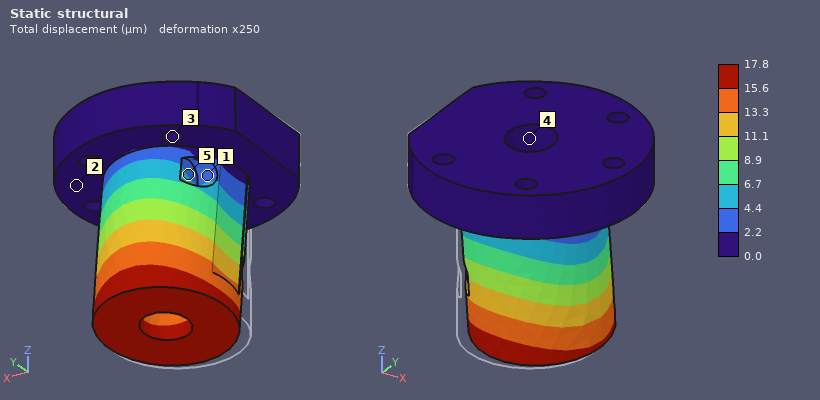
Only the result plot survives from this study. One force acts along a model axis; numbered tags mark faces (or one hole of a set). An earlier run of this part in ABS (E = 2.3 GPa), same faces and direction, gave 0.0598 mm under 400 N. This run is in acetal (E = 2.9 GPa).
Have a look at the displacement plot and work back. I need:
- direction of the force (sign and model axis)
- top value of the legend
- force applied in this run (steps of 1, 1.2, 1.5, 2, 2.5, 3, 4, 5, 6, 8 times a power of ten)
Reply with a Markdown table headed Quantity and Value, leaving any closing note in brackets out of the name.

| Quantity | Value |
|---|---|
| direction of the force | +Y |
| top value of the legend | 17.8 µm |
| force applied in this run | 150 N |
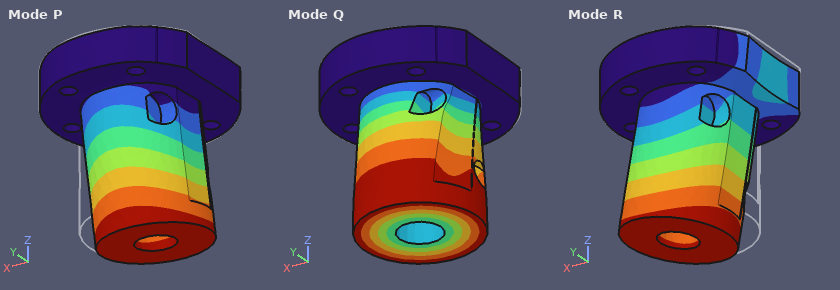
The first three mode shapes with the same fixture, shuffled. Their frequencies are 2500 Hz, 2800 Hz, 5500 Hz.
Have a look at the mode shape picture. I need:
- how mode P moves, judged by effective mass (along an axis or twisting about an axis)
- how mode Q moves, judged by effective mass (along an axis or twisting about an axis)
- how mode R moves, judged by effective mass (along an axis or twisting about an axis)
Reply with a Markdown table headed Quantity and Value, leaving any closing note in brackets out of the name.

| Quantity | Value |
|---|---|
| how mode P moves, judged by effective mass | along Y |
| how mode Q moves, judged by effective mass | twisting about Z |
| how mode R moves, judged by effective mass | along X |
